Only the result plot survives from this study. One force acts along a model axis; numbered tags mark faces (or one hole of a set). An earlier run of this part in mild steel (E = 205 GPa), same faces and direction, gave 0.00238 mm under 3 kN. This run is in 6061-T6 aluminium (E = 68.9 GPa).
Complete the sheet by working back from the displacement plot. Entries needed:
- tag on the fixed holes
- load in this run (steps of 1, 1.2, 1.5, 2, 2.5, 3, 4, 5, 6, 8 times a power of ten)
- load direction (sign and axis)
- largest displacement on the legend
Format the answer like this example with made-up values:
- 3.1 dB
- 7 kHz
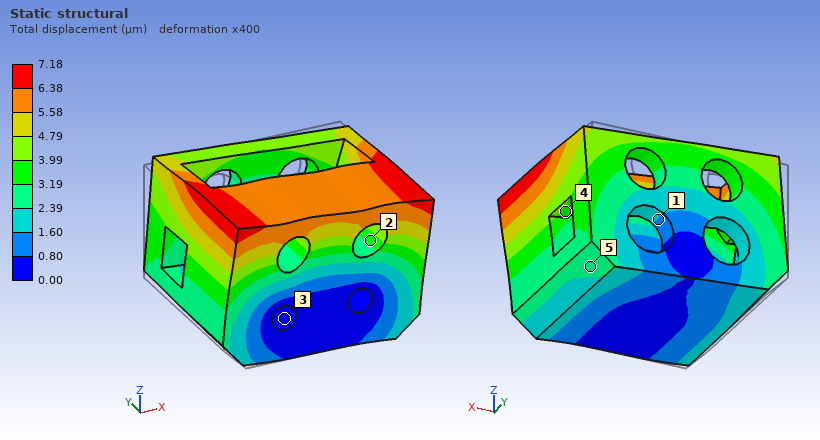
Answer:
- 3
- 3 kN
- +X
- 7.18 µm
